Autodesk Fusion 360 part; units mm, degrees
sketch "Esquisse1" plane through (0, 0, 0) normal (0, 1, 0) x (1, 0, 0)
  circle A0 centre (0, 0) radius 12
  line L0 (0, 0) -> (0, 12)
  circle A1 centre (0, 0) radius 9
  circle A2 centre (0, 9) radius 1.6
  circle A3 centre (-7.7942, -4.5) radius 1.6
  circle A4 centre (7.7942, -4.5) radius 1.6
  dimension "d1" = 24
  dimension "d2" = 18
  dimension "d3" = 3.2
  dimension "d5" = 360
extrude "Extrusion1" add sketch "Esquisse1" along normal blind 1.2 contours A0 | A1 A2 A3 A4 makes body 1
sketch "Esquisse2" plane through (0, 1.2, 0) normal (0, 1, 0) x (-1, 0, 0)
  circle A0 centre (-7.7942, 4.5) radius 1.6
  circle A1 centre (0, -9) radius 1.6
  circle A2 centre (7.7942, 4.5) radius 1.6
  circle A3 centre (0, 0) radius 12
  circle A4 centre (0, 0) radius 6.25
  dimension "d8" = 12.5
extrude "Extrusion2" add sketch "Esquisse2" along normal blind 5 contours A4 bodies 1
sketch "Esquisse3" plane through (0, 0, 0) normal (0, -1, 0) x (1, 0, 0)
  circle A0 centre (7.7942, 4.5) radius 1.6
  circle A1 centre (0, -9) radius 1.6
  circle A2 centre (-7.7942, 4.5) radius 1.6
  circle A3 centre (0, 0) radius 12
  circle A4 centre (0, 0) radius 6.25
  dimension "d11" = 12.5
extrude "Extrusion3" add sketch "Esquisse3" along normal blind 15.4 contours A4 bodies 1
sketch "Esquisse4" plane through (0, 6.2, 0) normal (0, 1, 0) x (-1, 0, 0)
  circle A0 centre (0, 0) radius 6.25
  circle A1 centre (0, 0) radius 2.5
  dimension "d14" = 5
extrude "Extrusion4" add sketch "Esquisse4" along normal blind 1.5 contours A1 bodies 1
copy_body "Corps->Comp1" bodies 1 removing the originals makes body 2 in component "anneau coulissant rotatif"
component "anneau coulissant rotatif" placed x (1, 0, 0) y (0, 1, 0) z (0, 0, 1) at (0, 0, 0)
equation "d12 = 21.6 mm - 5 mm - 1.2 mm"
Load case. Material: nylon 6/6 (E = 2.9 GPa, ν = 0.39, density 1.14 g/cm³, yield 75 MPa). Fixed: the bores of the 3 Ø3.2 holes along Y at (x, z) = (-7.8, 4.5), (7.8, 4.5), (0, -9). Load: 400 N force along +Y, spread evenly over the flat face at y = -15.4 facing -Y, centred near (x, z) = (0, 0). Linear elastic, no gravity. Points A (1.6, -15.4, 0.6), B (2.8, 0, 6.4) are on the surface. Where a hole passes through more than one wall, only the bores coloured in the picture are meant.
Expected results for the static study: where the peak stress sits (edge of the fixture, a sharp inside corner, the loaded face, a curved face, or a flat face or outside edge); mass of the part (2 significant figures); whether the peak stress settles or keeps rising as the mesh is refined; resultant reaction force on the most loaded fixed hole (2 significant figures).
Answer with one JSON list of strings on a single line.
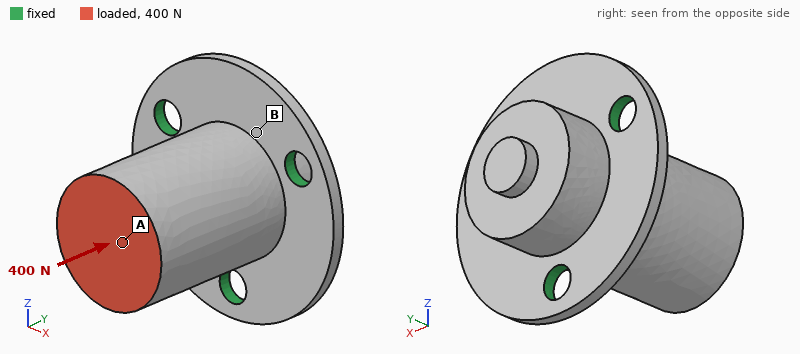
["edge of the fixture", "3.5 g", "keeps rising", "130 N"]
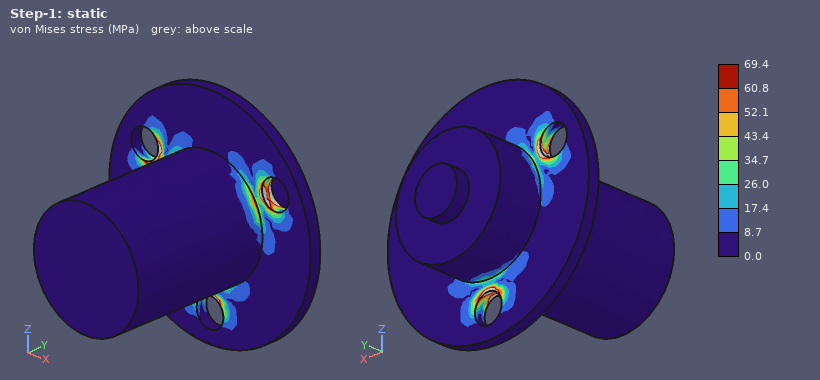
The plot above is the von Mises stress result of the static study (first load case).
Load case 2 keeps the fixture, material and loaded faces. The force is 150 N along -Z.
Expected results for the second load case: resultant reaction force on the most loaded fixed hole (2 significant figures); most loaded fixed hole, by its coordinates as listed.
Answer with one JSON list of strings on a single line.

["220 N", "(0, -9)"]
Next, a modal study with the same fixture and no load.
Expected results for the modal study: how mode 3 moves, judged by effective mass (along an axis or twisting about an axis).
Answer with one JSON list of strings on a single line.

["along Y"]
